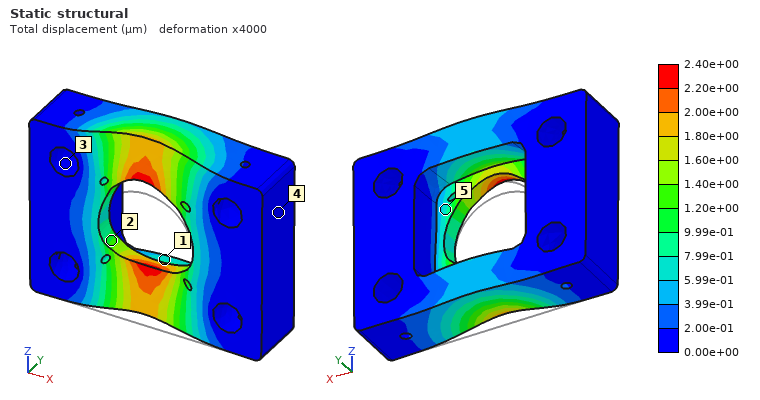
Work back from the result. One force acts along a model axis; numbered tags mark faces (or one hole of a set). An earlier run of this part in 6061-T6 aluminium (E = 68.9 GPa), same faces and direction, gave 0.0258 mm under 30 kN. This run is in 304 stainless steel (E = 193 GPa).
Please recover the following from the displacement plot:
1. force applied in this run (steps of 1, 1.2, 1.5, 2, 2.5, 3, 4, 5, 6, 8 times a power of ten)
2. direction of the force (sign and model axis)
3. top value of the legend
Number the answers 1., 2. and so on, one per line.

1. 8 kN
2. +Z
3. 2.40e+00 µm
